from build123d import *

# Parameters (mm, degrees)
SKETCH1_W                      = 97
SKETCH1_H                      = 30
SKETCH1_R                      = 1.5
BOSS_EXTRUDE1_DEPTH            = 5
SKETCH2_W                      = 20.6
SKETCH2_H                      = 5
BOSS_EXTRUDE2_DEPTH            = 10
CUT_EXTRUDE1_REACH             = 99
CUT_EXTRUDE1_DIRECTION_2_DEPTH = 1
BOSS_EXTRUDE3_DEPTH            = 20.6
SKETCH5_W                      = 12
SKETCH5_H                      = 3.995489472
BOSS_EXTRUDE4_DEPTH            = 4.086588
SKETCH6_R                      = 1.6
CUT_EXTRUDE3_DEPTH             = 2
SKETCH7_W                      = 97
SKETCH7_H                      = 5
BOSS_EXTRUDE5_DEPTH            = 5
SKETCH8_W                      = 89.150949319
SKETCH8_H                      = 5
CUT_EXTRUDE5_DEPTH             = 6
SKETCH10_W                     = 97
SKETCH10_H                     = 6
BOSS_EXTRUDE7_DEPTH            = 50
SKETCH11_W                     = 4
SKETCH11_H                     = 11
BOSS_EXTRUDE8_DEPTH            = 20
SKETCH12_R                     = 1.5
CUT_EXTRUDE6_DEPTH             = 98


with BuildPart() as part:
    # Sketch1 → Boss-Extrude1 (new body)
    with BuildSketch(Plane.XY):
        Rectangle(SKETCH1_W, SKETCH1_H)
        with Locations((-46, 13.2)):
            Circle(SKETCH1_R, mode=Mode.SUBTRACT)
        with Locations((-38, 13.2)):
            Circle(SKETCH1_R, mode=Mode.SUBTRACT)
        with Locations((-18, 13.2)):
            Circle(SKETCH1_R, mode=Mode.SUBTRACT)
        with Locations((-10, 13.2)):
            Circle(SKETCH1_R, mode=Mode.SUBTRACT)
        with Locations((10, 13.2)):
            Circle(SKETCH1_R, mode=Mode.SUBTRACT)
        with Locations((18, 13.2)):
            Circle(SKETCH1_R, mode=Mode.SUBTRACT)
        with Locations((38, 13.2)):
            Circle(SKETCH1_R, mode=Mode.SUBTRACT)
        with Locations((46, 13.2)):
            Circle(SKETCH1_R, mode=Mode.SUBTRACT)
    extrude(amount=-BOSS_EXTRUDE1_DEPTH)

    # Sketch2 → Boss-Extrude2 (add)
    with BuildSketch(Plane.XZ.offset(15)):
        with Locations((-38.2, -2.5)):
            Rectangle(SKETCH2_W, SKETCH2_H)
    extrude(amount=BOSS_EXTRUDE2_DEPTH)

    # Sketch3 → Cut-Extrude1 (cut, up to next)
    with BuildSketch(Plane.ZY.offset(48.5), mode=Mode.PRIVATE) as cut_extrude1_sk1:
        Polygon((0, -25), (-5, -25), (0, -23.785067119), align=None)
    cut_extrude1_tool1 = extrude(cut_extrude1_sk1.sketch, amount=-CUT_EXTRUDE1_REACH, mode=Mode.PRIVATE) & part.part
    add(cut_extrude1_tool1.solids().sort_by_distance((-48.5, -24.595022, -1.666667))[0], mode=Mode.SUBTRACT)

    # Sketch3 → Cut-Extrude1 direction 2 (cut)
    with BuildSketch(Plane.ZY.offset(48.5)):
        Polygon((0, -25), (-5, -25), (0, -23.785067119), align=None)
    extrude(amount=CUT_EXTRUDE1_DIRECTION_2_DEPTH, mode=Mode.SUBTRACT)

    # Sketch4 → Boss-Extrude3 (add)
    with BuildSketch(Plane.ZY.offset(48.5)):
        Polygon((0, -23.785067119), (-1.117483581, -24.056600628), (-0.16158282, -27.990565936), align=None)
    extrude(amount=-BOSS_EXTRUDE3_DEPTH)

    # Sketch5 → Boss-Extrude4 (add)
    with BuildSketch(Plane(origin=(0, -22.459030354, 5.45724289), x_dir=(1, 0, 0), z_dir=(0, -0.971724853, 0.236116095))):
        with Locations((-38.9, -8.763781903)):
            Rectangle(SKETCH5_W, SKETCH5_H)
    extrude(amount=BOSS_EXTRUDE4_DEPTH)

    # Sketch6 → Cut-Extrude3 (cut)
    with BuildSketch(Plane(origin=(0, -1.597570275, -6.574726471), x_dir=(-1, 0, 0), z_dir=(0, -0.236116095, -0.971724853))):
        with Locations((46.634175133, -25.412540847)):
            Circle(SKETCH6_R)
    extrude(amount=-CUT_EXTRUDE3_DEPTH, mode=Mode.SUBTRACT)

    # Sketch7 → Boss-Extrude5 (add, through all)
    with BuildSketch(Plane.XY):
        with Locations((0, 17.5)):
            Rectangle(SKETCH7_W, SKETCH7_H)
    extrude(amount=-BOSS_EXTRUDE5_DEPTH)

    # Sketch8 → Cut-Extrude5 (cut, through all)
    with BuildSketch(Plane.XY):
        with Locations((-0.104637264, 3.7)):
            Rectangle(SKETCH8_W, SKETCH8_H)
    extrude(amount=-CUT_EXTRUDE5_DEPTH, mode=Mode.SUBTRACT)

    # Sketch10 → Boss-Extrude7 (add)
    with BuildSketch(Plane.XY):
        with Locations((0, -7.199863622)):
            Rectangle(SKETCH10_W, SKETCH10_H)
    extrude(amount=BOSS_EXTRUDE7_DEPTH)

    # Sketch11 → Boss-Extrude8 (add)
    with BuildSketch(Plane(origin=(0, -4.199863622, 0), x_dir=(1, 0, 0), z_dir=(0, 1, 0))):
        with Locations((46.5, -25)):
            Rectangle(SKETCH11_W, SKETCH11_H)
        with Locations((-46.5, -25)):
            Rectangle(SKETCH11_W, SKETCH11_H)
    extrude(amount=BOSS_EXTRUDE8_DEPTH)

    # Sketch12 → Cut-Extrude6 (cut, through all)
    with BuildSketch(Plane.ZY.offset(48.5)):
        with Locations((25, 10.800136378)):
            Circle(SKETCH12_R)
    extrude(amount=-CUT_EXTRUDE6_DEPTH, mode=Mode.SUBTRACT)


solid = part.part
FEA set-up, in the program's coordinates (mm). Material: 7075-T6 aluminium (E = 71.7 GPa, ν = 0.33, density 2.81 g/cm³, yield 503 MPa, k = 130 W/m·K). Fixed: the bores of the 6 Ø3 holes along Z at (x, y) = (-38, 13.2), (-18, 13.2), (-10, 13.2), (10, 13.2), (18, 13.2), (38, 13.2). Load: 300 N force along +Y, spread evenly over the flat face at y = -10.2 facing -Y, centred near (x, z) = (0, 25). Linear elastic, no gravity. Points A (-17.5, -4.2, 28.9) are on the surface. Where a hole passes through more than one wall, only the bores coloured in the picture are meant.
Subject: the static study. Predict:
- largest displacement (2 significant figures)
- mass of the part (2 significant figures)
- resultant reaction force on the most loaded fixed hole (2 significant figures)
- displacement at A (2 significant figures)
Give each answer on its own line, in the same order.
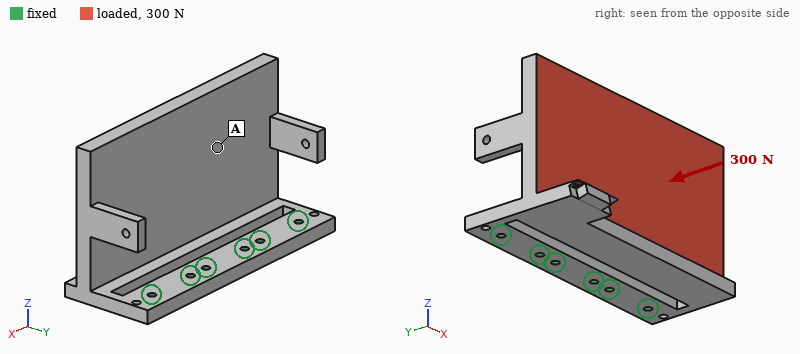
1.2 mm
130 g
200 N
0.74 mm
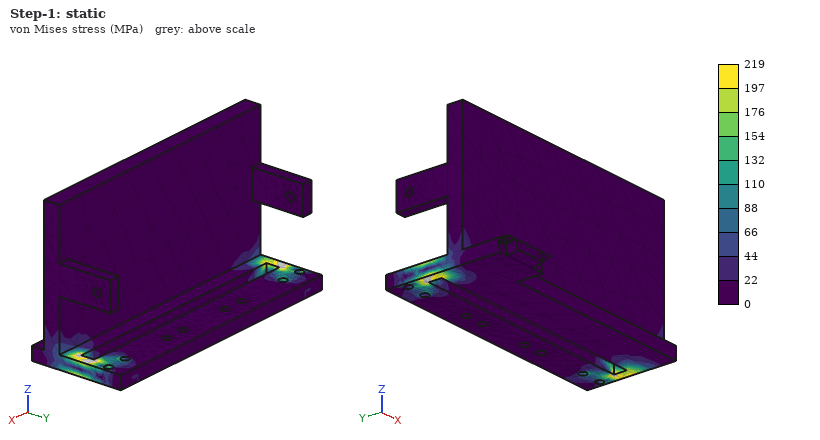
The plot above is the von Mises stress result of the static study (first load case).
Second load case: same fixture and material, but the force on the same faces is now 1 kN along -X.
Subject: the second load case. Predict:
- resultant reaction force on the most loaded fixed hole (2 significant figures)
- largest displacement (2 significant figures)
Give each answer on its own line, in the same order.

640 N
0.15 mm
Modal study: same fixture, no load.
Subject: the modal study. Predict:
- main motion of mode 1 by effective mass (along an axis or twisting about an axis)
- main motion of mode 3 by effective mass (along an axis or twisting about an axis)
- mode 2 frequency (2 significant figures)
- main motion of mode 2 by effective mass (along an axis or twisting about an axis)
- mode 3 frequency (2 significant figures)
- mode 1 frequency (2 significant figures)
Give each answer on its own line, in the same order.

along Y
along Z
1300 Hz
along X
1500 Hz
310 Hz
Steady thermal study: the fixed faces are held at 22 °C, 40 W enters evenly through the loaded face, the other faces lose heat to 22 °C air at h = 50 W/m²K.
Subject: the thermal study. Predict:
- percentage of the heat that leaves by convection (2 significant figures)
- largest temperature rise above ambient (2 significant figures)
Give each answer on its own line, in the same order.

66 %
51 K
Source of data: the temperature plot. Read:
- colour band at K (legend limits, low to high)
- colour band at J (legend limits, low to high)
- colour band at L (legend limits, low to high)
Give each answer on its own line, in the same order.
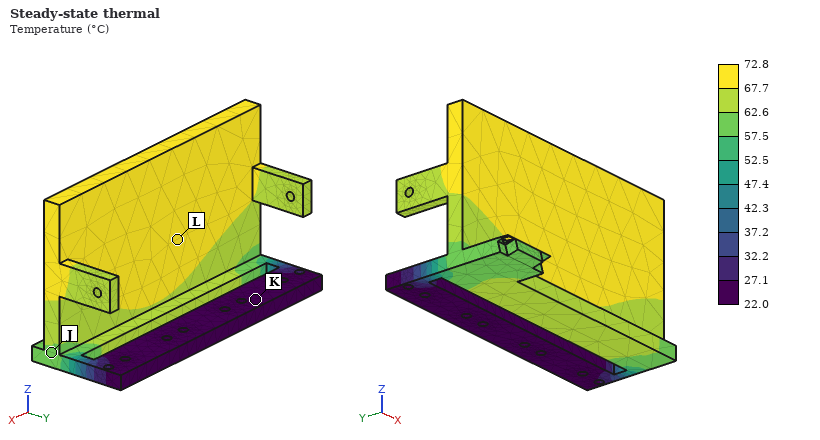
22.0 to 27.1 °C
57.5 to 62.6 °C
67.7 to 72.8 °C
